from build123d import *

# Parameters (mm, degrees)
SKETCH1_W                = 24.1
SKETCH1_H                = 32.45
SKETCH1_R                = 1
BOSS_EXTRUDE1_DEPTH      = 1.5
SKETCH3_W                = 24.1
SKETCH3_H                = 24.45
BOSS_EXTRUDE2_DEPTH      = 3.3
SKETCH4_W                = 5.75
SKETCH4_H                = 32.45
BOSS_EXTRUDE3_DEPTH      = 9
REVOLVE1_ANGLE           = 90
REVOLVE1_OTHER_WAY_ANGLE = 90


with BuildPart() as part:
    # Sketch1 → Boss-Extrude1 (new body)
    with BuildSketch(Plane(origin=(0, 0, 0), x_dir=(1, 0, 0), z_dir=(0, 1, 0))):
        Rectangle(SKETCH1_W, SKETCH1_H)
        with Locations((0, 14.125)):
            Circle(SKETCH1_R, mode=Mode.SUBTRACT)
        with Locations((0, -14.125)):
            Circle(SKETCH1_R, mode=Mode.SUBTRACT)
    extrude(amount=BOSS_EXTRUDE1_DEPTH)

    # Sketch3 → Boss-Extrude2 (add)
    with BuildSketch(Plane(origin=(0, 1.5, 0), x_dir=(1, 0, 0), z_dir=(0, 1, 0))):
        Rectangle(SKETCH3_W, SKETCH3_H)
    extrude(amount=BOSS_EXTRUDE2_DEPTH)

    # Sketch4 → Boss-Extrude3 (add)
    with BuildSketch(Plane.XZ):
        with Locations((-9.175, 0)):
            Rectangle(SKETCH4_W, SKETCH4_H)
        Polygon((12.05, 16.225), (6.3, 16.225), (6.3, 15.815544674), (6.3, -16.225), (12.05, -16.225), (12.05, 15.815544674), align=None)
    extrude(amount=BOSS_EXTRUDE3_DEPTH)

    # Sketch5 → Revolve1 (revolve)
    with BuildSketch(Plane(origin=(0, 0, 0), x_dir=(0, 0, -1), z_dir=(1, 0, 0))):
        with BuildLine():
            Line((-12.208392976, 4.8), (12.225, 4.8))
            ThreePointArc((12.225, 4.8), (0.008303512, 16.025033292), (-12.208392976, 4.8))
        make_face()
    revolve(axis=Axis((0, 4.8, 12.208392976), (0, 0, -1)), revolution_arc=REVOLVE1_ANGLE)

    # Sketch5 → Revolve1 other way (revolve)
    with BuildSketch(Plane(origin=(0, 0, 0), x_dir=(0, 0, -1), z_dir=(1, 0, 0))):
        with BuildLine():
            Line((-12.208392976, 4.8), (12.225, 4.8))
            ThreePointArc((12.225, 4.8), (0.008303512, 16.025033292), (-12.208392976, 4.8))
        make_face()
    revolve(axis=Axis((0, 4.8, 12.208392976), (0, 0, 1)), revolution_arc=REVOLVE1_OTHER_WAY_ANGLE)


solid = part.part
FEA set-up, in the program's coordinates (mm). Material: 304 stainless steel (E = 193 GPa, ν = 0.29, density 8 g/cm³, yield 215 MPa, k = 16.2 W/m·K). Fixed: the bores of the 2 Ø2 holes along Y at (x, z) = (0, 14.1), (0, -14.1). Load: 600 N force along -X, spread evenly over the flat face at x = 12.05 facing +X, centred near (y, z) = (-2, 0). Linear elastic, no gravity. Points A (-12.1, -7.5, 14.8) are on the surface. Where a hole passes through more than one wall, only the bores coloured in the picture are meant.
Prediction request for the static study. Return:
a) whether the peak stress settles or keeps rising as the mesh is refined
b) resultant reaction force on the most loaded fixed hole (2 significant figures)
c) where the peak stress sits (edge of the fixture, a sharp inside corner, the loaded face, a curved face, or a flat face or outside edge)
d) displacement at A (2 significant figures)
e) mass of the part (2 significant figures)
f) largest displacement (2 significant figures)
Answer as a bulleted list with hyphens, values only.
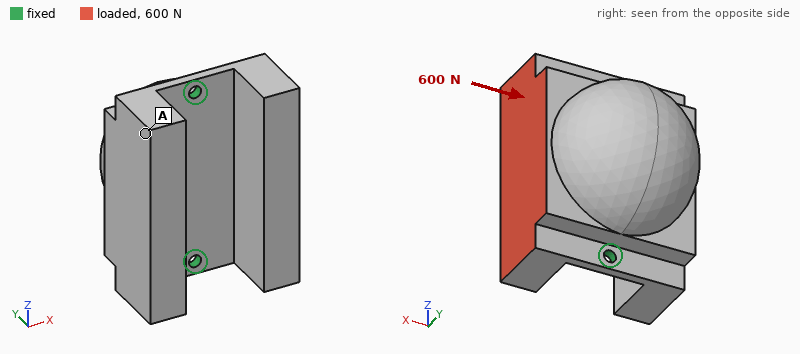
- keeps rising
- 300 N
- edge of the fixture
- 27 µm
- 77 g
- 32 µm
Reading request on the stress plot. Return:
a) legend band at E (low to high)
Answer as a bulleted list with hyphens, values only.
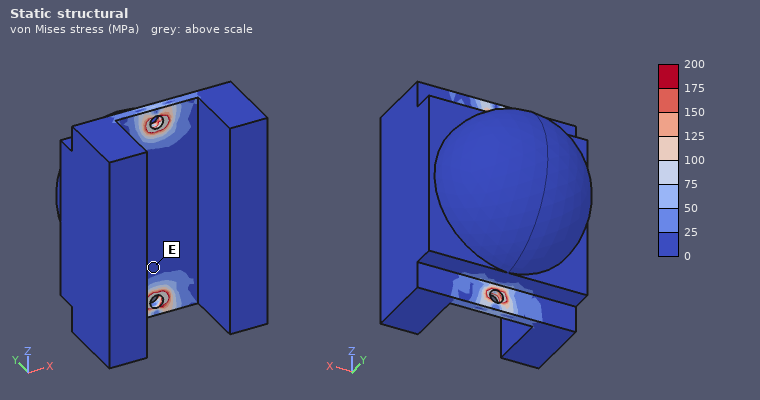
- 0 to 25 MPa
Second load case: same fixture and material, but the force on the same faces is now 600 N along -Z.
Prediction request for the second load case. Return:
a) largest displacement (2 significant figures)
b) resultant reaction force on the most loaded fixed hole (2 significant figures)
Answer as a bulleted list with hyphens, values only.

- 3.9 µm
- 400 N
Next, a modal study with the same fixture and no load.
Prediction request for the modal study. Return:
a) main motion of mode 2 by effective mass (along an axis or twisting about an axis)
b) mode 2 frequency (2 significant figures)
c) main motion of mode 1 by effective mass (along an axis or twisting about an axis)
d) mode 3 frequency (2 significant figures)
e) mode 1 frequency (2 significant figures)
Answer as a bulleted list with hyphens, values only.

- along Y
- 9300 Hz
- twisting about Z
- 12 kHz
- 1900 Hz
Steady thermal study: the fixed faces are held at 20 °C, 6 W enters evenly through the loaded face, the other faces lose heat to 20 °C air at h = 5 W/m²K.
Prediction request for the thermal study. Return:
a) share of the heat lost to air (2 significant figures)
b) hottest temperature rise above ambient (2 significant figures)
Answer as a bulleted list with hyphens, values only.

- 11 %
- 60 K
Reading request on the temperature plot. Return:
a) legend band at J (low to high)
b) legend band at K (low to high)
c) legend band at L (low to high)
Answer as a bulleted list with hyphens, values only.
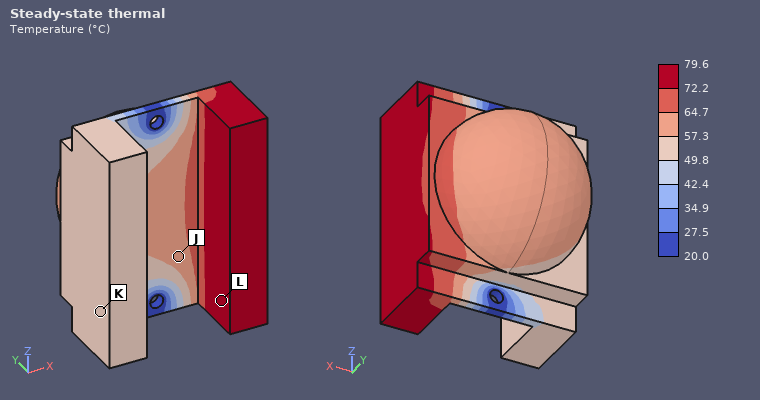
- 57.3 to 64.7 °C
- 49.8 to 57.3 °C
- 72.2 to 79.6 °C
